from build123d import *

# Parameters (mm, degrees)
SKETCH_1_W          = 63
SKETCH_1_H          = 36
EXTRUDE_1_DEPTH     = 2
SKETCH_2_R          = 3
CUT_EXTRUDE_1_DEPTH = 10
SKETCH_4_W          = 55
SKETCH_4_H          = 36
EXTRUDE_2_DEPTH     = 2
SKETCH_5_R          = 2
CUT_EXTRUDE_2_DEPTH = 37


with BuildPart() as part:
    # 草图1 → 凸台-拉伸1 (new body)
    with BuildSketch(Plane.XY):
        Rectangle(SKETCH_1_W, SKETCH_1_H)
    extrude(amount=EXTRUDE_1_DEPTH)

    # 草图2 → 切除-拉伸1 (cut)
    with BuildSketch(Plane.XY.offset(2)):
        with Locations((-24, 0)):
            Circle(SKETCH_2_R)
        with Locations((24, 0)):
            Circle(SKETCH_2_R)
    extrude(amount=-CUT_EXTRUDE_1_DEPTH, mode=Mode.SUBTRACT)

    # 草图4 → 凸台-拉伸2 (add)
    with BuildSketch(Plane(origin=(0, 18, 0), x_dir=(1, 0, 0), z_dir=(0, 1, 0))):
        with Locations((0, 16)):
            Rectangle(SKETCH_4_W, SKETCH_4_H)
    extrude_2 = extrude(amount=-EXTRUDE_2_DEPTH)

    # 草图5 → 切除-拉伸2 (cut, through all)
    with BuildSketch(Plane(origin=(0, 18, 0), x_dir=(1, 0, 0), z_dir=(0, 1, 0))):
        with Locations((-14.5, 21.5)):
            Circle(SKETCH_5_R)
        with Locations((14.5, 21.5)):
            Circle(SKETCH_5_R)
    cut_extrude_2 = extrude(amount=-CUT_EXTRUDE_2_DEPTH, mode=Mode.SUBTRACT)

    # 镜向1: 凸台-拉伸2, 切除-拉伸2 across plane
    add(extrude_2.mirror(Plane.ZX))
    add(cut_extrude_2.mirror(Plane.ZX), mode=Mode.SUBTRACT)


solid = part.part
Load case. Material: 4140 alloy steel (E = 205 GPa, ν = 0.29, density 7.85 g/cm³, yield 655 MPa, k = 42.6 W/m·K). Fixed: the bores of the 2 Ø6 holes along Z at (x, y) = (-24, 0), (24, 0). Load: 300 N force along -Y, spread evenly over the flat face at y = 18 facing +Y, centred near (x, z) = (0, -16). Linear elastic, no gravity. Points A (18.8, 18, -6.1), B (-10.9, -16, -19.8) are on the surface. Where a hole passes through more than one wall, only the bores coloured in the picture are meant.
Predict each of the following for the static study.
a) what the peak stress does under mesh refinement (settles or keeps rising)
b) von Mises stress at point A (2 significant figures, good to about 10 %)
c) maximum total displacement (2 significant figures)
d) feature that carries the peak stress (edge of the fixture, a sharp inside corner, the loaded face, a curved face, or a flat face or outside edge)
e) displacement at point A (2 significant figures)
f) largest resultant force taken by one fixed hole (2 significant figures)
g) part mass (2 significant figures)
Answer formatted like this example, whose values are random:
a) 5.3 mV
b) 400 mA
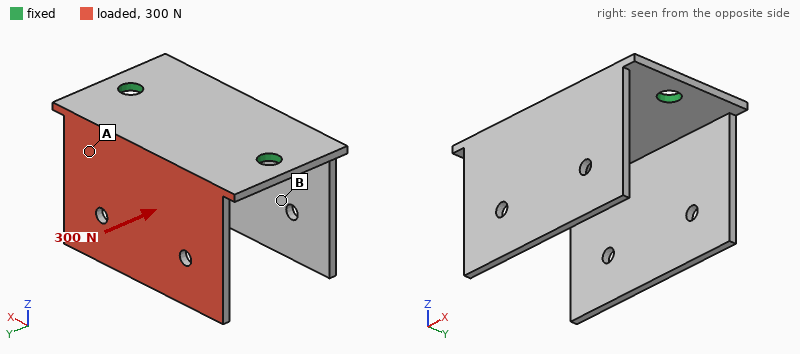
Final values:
a) keeps rising
b) 74 MPa
c) 0.50 mm
d) edge of the fixture
e) 0.12 mm
f) 150 N
g) 93 g
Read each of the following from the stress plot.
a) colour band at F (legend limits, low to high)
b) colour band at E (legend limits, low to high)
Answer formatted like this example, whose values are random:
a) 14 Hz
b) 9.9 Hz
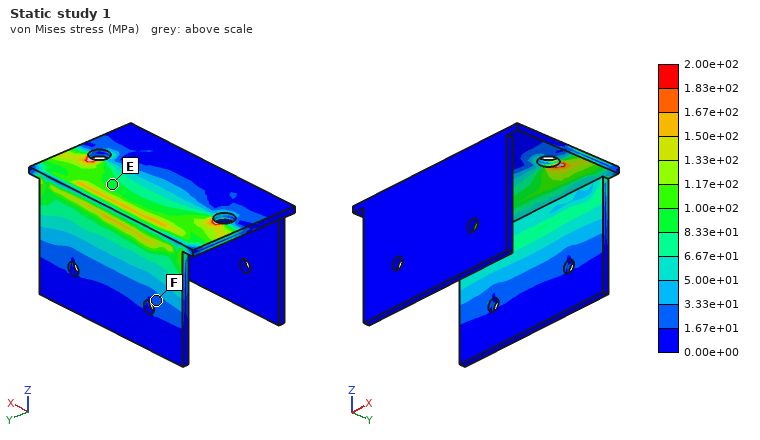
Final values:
a) 1.67e+01 to 3.33e+01 MPa
b) 8.33e+01 to 1.00e+02 MPa
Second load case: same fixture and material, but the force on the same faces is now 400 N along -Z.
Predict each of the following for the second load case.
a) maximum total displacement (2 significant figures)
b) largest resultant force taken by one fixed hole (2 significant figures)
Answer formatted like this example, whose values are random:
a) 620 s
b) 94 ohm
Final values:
a) 0.27 mm
b) 200 N
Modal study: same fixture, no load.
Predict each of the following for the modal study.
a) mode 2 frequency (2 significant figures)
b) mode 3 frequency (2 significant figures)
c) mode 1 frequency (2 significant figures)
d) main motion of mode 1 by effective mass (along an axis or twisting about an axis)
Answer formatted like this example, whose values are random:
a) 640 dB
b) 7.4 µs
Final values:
a) 850 Hz
b) 1800 Hz
c) 810 Hz
d) along Y
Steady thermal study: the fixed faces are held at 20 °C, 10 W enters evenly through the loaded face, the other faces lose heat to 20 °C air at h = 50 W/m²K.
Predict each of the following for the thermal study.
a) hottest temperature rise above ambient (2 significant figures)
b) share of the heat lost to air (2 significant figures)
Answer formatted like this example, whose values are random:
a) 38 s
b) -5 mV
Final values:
a) 40 K
b) 57 %
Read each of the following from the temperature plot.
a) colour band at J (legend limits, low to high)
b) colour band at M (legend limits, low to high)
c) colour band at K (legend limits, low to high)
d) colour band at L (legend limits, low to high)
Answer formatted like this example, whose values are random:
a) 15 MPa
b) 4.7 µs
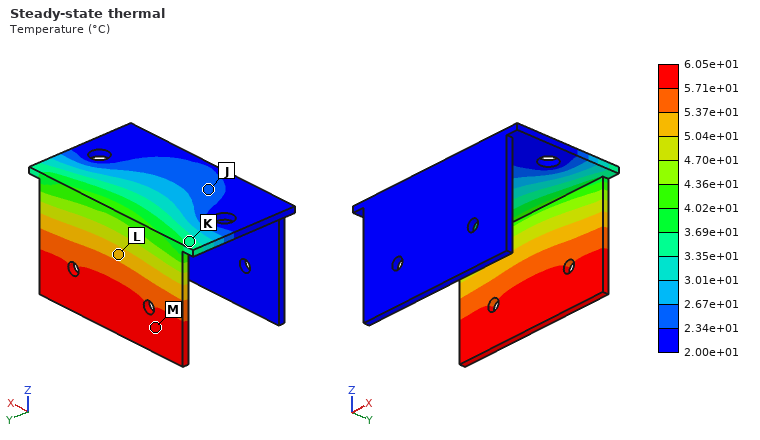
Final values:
a) 2.34e+01 to 2.67e+01 °C
b) 5.71e+01 to 6.05e+01 °C
c) 3.35e+01 to 3.69e+01 °C
d) 5.04e+01 to 5.37e+01 °C
